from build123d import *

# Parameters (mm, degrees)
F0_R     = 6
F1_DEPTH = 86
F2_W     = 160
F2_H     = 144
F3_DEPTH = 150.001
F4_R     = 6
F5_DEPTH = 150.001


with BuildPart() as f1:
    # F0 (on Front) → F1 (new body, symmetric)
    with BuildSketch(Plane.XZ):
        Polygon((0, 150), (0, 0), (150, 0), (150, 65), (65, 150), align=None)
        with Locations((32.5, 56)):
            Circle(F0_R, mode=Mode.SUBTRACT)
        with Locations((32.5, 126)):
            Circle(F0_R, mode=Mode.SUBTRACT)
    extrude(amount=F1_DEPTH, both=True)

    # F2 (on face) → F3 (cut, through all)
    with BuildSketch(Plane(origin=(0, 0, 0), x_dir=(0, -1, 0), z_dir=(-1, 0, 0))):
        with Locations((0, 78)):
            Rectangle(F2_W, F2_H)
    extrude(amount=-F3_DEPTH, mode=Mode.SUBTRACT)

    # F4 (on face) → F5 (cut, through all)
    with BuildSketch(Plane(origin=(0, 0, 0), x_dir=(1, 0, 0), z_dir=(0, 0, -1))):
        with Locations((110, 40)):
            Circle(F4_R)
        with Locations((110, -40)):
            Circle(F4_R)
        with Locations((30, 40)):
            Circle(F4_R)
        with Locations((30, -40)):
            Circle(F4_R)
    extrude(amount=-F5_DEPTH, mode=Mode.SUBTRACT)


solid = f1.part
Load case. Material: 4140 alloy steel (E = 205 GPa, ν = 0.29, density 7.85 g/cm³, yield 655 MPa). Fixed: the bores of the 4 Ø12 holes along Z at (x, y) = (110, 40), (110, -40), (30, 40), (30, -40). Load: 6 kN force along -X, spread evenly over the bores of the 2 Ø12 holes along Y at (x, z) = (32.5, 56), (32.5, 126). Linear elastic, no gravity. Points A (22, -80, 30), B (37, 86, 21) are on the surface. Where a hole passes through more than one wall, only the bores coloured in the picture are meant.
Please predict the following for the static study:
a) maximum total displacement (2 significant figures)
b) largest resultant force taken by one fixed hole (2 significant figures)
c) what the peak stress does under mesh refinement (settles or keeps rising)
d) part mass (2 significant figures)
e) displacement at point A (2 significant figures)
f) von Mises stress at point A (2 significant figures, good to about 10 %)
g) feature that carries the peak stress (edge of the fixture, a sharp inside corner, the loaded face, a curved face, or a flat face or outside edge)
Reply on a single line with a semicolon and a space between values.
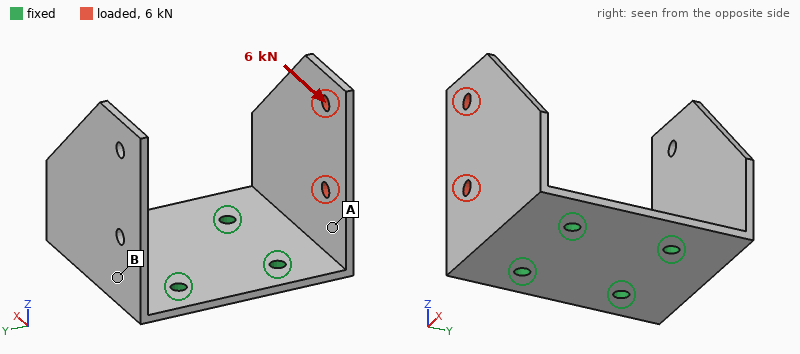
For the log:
1.2 mm; 7.1 kN; keeps rising; 2.9 kg; 0.40 mm; 110 MPa; edge of the fixture
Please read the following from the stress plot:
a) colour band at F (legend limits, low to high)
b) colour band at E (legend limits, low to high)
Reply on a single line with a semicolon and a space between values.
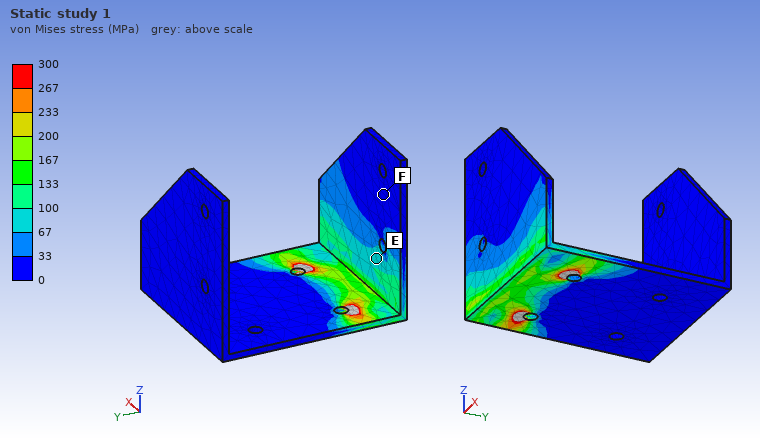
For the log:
0 to 33 MPa; 67 to 100 MPa
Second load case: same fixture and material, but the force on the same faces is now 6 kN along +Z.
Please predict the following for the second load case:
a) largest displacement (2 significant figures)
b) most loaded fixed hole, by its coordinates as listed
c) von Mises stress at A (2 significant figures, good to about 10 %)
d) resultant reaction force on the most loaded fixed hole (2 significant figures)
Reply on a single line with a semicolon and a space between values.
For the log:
1.7 mm; (30, -40); 59 MPa; 5.7 kN
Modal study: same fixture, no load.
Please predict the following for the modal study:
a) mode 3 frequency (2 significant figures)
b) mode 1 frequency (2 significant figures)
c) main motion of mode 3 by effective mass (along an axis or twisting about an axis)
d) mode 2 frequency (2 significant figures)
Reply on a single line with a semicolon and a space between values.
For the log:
520 Hz; 200 Hz; along X; 200 Hz
